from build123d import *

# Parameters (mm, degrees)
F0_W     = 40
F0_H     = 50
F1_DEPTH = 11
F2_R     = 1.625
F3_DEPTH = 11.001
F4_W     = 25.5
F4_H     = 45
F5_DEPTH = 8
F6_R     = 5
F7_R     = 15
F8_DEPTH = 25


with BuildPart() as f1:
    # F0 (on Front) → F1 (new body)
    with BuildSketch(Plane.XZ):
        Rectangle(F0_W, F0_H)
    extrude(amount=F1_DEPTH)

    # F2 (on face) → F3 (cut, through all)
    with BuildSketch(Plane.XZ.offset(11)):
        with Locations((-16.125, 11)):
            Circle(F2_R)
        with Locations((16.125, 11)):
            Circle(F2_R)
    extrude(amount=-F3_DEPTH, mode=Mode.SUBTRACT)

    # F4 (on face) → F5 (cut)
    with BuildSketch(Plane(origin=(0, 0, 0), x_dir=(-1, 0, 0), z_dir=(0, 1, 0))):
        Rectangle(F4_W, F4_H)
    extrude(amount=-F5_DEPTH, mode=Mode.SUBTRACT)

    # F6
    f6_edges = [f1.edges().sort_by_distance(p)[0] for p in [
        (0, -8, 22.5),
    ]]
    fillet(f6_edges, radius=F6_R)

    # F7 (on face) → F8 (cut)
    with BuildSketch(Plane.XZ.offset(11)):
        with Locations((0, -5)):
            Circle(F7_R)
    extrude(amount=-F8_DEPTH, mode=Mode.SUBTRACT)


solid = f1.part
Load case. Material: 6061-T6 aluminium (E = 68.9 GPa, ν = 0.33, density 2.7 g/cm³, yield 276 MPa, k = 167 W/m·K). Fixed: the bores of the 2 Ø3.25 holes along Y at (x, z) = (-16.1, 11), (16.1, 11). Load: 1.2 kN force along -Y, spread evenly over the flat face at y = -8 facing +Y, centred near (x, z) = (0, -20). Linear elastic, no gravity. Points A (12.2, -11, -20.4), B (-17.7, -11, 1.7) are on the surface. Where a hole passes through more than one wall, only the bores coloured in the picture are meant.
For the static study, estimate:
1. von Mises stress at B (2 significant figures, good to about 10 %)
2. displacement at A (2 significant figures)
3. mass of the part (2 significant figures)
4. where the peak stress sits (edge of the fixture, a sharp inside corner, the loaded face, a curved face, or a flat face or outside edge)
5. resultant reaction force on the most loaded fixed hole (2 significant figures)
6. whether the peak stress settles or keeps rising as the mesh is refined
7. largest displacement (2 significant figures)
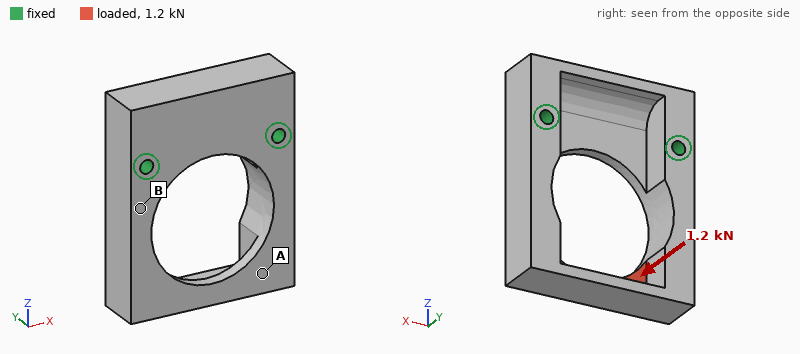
110 MPa
0.14 mm
28 g
edge of the fixture
600 N
keeps rising
0.18 mm
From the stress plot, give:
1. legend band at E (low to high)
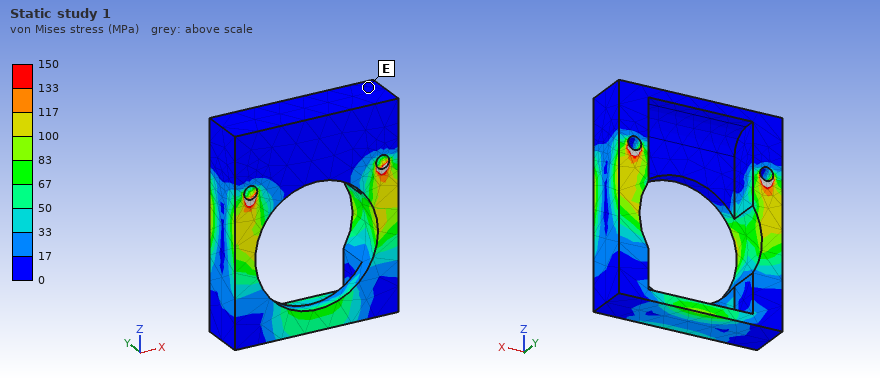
0 to 17 MPa
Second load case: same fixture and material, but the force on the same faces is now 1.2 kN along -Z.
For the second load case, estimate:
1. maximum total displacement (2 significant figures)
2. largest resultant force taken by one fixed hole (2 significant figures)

37 µm
650 N
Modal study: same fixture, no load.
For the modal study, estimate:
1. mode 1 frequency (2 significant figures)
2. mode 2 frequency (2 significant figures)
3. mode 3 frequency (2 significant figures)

5000 Hz
5200 Hz
7900 Hz
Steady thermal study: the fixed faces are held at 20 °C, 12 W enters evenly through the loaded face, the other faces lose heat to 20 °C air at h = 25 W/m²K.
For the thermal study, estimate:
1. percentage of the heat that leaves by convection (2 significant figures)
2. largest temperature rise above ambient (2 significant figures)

7.5 %
21 K
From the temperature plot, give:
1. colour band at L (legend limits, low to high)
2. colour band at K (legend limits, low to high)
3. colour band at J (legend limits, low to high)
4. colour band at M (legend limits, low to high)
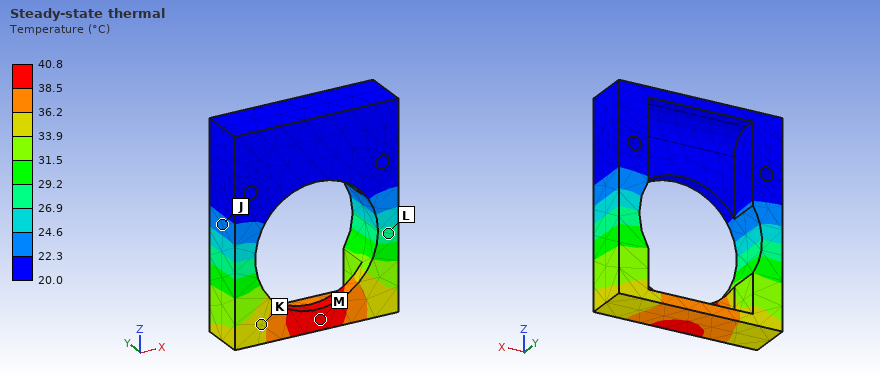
26.9 to 29.2 °C
33.9 to 36.2 °C
22.3 to 24.6 °C
38.5 to 40.8 °C
